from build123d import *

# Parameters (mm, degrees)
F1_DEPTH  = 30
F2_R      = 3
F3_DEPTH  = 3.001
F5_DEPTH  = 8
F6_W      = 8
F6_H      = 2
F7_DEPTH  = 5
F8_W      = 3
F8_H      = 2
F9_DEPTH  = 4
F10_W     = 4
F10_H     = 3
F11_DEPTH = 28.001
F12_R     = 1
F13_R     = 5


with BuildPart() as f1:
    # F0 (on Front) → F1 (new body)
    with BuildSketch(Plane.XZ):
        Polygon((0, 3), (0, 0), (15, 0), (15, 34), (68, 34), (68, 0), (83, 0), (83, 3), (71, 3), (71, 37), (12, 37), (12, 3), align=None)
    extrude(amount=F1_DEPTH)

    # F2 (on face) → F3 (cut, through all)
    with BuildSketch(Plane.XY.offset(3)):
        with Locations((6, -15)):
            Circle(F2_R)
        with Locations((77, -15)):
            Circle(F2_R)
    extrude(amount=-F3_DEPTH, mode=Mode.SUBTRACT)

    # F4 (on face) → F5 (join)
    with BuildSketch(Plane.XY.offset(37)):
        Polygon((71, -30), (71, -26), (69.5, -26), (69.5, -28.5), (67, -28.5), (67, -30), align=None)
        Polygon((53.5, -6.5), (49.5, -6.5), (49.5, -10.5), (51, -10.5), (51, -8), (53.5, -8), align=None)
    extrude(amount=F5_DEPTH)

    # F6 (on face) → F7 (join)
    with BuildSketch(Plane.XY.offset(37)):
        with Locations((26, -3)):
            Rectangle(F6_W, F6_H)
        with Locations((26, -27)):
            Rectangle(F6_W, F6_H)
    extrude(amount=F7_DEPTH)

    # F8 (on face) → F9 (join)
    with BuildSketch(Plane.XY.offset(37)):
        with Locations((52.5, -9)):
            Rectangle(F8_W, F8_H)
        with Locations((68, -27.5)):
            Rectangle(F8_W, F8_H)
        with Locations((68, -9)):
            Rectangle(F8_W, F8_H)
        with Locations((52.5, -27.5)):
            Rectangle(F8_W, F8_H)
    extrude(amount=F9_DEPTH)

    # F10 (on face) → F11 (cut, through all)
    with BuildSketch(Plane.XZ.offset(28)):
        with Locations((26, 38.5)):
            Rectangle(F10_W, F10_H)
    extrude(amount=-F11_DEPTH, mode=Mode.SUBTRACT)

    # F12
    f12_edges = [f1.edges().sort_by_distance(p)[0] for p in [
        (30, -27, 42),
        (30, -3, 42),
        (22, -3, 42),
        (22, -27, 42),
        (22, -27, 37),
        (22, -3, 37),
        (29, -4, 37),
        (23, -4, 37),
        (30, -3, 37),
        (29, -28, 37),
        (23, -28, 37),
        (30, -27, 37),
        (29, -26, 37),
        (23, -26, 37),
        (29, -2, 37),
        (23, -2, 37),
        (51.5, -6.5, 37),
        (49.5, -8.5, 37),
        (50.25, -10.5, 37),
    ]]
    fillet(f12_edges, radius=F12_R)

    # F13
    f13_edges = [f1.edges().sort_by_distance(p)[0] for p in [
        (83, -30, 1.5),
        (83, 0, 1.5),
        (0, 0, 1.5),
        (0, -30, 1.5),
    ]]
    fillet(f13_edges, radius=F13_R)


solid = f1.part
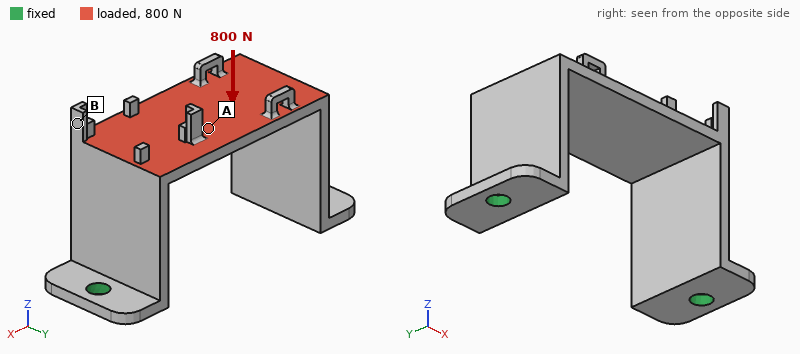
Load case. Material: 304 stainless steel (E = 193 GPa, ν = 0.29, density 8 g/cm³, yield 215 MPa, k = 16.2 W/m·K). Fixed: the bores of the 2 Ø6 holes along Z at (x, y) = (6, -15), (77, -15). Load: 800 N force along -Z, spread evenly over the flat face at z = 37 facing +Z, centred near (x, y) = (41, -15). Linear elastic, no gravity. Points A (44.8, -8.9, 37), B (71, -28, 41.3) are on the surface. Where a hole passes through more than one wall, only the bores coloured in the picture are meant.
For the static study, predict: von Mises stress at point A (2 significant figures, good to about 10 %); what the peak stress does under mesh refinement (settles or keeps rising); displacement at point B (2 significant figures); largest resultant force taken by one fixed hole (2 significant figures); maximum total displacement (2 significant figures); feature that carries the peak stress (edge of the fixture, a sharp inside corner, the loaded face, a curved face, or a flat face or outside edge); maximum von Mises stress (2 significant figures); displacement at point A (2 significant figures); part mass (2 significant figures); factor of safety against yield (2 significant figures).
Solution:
53 MPa
settles
11 µm
420 N
52 µm
the loaded face
72 MPa
47 µm
110 g
3.0
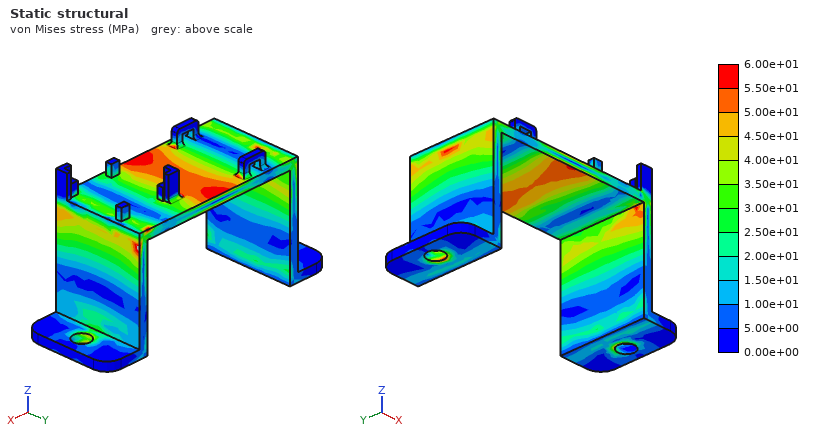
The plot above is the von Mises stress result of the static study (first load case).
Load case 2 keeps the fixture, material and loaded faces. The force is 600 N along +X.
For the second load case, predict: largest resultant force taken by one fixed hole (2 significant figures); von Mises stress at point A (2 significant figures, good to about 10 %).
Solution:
360 N
12 MPa
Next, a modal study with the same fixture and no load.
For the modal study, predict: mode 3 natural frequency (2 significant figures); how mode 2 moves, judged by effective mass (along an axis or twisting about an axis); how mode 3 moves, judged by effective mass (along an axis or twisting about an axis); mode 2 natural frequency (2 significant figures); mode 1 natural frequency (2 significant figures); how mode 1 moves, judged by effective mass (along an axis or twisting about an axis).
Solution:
2300 Hz
along Y
twisting about Z
1600 Hz
1300 Hz
along X
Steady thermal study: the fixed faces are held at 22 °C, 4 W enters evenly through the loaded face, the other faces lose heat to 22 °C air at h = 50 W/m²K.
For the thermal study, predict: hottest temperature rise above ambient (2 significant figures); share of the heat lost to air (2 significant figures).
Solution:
20 K
88 %
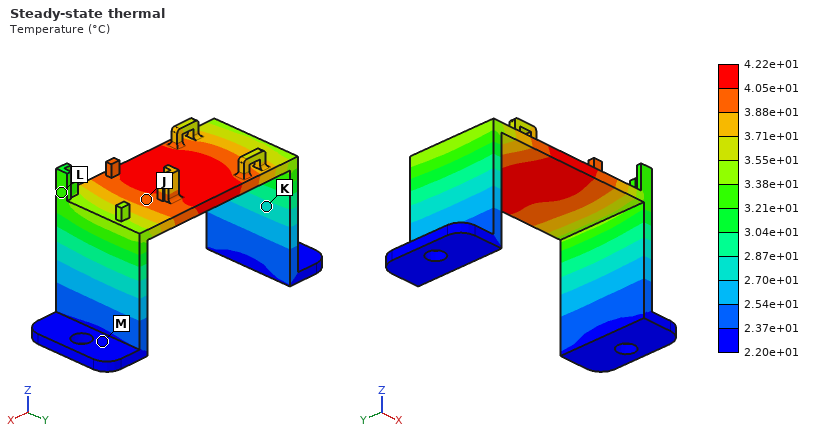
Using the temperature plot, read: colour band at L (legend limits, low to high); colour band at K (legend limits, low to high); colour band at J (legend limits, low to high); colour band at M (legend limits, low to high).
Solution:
3.21e+01 to 3.38e+01 °C
2.70e+01 to 2.87e+01 °C
3.88e+01 to 4.05e+01 °C
2.20e+01 to 2.37e+01 °C
